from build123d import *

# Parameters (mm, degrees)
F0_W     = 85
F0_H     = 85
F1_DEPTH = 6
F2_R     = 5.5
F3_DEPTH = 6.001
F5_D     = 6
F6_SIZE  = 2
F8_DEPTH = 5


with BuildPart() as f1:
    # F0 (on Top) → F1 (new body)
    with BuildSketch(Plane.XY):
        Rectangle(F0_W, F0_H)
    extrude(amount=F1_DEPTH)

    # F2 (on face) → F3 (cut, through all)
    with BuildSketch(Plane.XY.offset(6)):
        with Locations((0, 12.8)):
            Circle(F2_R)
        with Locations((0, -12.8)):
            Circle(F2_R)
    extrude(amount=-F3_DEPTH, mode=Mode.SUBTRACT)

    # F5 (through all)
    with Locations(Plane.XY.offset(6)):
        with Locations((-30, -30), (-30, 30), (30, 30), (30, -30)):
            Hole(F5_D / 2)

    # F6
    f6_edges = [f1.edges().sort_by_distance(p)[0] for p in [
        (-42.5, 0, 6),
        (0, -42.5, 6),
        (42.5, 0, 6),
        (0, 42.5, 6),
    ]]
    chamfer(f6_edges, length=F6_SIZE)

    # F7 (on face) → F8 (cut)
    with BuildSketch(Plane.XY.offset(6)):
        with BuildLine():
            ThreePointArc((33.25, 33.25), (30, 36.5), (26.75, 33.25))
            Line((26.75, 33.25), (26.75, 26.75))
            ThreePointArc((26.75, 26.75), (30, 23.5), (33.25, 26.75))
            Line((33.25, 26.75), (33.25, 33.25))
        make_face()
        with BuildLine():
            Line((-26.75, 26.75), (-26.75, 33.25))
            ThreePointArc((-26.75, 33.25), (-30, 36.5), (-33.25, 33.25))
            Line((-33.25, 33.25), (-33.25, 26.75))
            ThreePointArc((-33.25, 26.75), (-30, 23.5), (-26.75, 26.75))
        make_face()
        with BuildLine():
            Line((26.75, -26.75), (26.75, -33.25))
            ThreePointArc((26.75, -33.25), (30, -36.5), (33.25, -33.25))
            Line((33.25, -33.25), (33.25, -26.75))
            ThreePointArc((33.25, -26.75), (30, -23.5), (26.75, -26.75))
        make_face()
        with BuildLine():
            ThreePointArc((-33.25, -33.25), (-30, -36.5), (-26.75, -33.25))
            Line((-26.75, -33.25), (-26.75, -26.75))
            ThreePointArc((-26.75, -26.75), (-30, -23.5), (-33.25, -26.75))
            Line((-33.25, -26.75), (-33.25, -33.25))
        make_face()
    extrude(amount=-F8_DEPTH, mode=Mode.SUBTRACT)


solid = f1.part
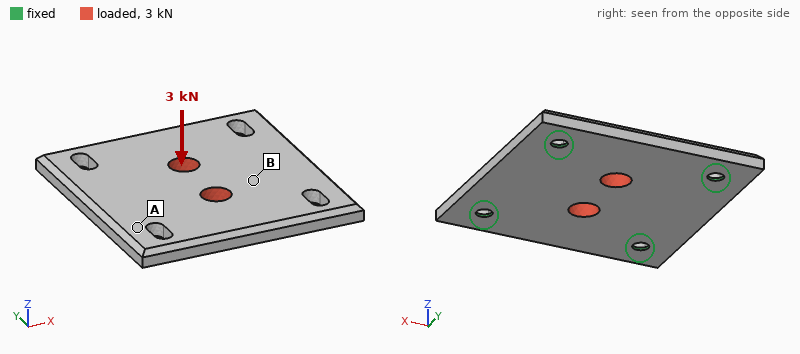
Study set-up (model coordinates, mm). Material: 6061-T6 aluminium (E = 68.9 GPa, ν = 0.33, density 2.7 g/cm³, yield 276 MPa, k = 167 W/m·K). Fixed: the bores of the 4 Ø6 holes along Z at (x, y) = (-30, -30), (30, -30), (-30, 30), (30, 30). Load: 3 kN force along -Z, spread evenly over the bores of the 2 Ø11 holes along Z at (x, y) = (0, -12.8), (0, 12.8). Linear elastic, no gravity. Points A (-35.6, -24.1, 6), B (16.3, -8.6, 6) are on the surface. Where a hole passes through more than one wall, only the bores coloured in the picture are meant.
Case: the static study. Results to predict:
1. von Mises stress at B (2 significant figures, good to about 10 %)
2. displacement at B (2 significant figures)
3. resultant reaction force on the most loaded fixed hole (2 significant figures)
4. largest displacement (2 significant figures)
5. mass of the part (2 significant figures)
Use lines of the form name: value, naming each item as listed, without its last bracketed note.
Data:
von Mises stress at B: 40 MPa
displacement at B: 0.097 mm
resultant reaction force on the most loaded fixed hole: 2.1 kN
largest displacement: 0.15 mm
mass of the part: 110 g
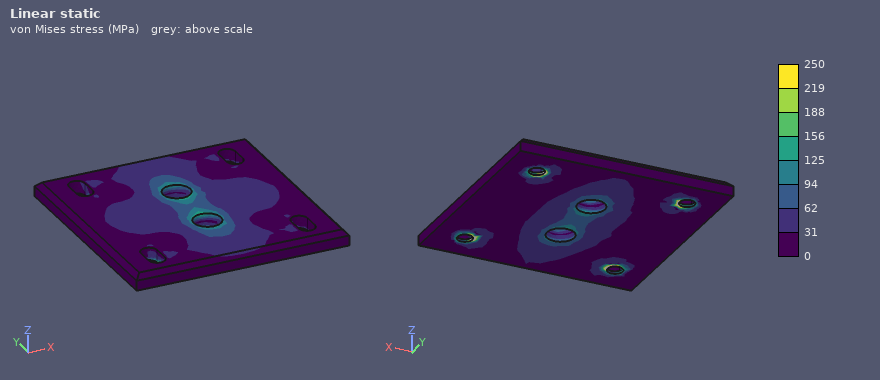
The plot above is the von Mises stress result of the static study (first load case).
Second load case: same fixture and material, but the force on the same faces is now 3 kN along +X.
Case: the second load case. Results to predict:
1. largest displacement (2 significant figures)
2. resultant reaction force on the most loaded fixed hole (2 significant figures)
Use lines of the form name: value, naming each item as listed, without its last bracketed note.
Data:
largest displacement: 7.1 µm
resultant reaction force on the most loaded fixed hole: 770 N
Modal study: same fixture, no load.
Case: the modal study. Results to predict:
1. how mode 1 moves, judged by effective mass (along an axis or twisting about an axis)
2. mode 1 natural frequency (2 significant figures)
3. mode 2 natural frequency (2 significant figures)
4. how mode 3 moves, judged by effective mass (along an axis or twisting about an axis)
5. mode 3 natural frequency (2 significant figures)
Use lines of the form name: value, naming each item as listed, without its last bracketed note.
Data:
how mode 1 moves, judged by effective mass: along Z
mode 1 natural frequency: 4400 Hz
mode 2 natural frequency: 5800 Hz
how mode 3 moves, judged by effective mass: twisting about Y
mode 3 natural frequency: 6200 Hz
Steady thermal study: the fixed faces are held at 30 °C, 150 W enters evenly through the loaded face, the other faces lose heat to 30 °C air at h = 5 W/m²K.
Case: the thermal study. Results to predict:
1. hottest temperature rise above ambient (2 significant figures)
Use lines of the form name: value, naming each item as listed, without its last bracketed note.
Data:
hottest temperature rise above ambient: 64 K
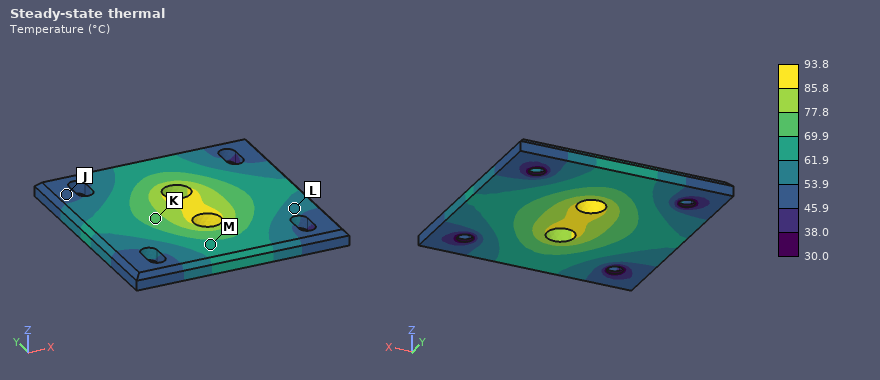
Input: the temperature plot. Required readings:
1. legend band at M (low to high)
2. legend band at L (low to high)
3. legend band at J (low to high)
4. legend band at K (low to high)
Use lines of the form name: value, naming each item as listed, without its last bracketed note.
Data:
legend band at M: 61.9 to 69.9 °C
legend band at L: 53.9 to 61.9 °C
legend band at J: 45.9 to 53.9 °C
legend band at K: 69.9 to 77.8 °C
